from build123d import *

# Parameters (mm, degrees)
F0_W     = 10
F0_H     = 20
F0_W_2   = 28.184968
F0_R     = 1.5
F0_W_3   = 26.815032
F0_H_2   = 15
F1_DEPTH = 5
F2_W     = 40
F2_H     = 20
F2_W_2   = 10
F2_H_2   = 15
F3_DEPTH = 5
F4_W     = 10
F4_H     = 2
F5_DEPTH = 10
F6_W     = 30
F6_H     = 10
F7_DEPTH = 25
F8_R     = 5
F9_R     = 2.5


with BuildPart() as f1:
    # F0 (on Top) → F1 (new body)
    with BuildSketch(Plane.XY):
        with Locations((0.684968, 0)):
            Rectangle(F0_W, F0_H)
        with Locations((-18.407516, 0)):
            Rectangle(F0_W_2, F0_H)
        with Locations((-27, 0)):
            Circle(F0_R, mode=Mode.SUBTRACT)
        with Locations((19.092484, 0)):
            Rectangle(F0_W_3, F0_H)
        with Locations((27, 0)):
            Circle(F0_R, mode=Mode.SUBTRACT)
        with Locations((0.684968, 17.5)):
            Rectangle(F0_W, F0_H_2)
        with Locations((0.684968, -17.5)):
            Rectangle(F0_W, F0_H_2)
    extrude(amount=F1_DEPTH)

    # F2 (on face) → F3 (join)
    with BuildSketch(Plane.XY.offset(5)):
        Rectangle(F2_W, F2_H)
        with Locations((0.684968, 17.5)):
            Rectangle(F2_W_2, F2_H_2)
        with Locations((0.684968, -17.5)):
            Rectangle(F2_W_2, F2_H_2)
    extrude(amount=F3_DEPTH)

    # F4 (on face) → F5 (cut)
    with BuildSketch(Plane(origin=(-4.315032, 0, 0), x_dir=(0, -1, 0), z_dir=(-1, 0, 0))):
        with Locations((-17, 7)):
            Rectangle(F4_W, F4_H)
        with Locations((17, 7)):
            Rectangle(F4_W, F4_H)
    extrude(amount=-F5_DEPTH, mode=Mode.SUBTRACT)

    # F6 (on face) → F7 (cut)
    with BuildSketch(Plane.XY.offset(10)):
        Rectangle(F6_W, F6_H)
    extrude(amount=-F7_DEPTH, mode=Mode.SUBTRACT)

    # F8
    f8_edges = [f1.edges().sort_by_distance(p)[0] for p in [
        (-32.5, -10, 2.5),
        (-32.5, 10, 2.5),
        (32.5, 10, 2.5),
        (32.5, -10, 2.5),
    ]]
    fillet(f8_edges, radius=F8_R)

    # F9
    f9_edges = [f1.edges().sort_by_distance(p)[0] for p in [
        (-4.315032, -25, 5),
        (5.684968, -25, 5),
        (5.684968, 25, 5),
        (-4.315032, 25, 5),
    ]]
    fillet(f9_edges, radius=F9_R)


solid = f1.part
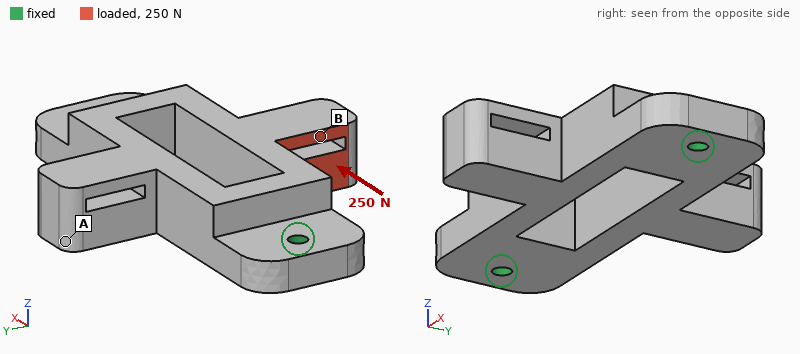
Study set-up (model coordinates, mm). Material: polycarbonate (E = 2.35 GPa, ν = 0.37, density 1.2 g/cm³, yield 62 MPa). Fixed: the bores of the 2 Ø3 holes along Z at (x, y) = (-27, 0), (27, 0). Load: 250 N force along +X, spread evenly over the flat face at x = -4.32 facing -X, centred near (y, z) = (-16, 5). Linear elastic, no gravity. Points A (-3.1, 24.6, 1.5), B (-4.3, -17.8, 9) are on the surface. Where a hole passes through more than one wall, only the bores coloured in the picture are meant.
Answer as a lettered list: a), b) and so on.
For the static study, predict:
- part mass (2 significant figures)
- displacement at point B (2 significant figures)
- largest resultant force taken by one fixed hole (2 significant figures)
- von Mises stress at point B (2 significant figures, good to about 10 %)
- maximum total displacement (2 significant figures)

a) 12 g
b) 0.20 mm
c) 150 N
d) 3.1 MPa
e) 0.31 mm
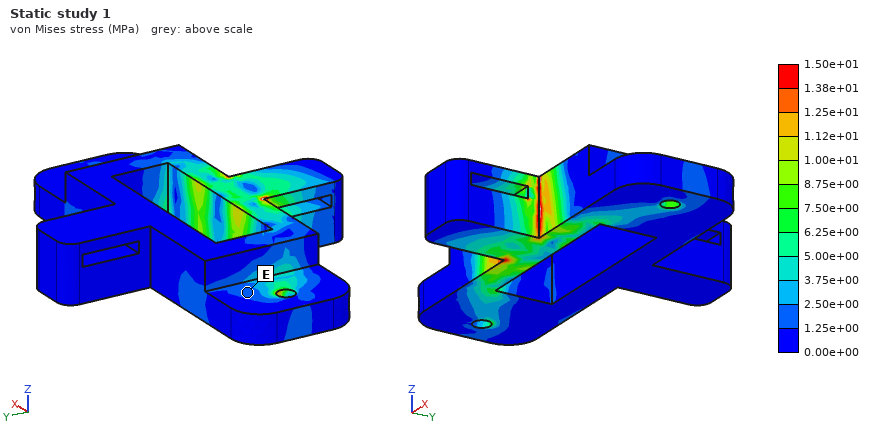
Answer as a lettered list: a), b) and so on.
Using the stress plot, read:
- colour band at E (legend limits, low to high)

a) 1.25e+00 to 2.50e+00 MPa
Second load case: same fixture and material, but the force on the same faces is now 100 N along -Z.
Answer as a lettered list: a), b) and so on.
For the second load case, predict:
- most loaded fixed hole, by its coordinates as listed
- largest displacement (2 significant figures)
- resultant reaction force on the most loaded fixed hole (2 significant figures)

a) (-27, 0)
b) 0.90 mm
c) 88 N
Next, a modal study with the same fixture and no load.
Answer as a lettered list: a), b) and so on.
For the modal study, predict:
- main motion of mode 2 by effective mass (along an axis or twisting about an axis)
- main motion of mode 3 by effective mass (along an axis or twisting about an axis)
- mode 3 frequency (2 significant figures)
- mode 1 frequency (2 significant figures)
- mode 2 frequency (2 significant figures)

a) along Z
b) along Y
c) 2800 Hz
d) 1200 Hz
e) 1600 Hz
